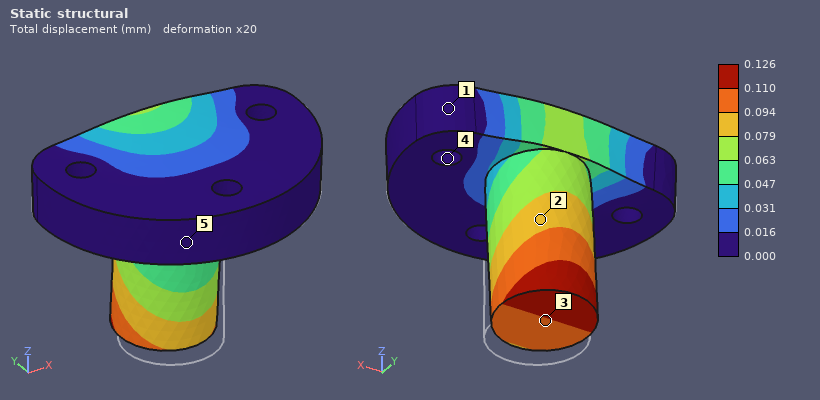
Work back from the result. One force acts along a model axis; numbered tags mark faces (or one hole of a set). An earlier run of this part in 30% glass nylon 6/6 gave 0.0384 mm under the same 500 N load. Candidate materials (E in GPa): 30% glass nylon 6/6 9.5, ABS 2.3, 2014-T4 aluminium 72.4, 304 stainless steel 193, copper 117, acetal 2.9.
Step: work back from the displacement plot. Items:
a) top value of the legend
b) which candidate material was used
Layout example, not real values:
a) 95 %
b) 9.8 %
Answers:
a) 0.126 mm
b) acetal
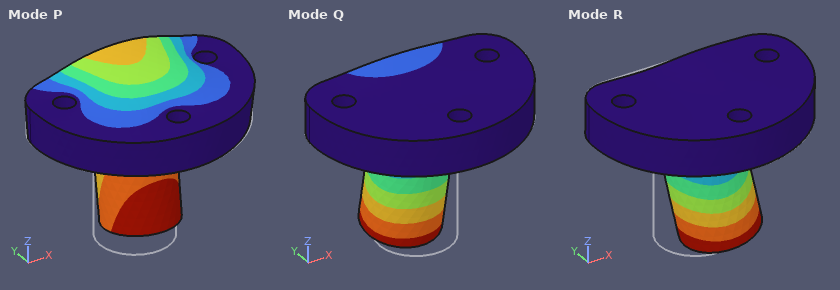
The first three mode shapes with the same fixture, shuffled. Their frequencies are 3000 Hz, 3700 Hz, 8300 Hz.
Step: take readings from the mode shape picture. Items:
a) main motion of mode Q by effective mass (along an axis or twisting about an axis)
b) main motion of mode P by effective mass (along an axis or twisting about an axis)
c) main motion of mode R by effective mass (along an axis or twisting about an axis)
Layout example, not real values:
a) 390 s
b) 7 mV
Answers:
a) along Y
b) along Z
c) along X
